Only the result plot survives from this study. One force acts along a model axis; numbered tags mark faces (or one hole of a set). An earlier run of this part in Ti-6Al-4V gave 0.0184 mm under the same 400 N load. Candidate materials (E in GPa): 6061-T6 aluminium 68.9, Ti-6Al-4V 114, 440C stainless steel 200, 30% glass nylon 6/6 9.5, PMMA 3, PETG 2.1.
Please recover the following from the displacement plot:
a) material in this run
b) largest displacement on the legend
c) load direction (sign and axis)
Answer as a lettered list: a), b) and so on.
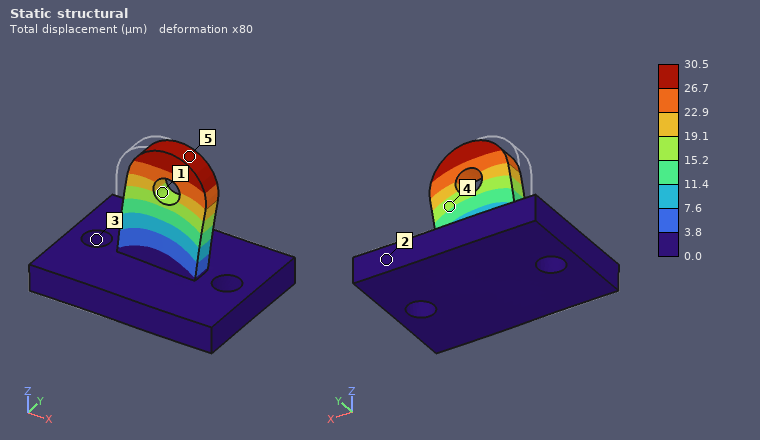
a) 6061-T6 aluminium
b) 30.5 µm
c) +X
